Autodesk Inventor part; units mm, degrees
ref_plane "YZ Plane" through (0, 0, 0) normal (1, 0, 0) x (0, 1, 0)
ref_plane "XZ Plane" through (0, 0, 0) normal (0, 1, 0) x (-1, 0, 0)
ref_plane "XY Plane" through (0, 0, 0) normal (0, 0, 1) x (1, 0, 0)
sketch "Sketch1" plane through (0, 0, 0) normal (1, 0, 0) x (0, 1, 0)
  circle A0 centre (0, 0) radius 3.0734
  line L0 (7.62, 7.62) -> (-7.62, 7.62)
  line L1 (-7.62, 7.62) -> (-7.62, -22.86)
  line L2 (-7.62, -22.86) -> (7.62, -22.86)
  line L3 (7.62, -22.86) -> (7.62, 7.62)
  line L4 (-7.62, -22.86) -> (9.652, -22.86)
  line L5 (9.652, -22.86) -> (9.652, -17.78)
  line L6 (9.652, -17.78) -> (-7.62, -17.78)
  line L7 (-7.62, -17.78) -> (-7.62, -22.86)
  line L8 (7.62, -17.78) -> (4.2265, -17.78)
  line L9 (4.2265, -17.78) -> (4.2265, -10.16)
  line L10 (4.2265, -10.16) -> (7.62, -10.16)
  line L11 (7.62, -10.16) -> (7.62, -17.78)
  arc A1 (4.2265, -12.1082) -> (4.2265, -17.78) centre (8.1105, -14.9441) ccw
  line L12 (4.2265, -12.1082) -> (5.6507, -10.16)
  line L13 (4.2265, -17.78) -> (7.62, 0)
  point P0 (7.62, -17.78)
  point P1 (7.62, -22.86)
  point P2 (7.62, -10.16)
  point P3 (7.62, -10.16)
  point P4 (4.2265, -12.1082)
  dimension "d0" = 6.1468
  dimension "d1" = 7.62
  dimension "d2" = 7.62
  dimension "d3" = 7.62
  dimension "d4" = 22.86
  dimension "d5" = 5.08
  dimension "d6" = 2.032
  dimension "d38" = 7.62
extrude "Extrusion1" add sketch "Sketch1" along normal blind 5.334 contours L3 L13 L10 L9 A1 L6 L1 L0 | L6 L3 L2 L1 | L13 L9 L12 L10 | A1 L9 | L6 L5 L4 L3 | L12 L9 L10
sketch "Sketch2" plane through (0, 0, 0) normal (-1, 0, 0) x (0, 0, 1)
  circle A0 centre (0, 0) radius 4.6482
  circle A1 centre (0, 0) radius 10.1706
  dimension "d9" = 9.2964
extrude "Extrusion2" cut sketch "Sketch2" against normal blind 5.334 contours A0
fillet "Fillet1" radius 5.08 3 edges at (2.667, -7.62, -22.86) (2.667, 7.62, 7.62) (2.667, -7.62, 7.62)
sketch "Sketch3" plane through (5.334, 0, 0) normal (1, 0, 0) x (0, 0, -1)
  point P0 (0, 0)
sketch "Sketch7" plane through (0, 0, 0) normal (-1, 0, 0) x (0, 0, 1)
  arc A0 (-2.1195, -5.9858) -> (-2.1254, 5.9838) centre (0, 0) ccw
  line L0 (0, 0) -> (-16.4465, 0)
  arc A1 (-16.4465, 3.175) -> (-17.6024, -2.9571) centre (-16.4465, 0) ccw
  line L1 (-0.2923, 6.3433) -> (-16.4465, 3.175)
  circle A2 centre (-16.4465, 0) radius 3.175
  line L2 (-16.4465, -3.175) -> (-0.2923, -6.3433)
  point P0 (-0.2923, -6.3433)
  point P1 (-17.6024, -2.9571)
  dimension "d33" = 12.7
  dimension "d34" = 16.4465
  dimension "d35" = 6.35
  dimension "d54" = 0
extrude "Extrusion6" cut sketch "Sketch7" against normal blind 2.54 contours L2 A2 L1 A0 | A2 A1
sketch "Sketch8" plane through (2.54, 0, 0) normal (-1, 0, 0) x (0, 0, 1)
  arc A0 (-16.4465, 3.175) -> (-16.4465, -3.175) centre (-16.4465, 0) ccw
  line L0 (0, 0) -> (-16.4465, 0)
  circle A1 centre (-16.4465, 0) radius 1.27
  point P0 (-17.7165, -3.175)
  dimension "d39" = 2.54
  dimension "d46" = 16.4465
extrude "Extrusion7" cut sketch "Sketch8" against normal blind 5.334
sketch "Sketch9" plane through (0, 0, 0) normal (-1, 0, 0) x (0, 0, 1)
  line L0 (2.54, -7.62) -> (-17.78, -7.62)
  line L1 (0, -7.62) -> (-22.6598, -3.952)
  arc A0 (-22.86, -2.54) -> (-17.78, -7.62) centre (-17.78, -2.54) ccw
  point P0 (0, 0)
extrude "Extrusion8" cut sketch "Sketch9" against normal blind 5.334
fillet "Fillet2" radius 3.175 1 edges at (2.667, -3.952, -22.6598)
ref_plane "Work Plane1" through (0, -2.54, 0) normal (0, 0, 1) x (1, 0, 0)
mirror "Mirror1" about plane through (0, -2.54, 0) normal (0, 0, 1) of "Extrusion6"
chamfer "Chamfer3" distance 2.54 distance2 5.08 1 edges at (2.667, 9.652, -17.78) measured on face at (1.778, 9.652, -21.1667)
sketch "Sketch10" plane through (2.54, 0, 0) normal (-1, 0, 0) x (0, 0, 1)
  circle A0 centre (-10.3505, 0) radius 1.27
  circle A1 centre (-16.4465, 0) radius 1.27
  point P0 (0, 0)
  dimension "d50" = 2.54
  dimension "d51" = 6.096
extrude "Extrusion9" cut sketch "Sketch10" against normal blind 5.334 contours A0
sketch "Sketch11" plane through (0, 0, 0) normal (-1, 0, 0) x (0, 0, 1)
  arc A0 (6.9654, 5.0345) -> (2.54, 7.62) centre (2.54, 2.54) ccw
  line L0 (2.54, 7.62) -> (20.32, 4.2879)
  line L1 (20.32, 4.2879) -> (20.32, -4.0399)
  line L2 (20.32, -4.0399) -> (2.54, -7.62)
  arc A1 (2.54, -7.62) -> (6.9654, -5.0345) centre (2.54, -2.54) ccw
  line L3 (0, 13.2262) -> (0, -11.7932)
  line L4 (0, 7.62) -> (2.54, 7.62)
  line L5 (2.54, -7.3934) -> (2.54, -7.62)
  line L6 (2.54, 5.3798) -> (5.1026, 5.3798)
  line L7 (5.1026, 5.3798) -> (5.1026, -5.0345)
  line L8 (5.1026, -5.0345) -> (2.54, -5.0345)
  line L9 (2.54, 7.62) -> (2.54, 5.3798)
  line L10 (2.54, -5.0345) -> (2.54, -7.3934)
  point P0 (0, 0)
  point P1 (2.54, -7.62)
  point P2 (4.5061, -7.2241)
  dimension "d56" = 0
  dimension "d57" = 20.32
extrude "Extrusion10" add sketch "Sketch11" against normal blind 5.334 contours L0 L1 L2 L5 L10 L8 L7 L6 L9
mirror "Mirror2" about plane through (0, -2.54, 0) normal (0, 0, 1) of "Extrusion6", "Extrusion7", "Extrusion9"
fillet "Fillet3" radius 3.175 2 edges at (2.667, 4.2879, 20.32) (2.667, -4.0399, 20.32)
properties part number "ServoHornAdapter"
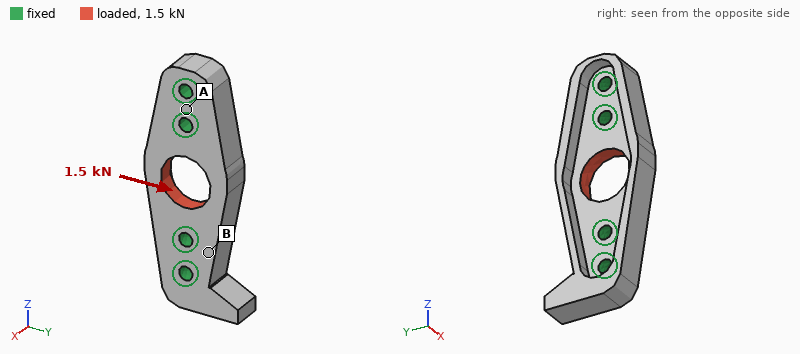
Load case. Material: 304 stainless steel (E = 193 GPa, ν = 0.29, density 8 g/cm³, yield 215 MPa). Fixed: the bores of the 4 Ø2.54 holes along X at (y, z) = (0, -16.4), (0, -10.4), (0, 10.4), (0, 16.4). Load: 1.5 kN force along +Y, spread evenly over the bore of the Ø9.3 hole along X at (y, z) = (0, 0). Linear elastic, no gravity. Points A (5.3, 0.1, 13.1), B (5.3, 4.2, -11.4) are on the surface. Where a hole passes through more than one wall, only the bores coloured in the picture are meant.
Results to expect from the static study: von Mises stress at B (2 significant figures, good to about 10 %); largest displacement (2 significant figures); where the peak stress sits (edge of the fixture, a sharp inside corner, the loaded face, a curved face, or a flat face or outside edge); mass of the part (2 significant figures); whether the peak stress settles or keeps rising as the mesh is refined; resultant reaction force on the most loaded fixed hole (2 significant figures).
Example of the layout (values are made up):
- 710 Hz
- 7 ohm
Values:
- 16 MPa
- 3.8 µm
- edge of the fixture
- 13 g
- keeps rising
- 850 N
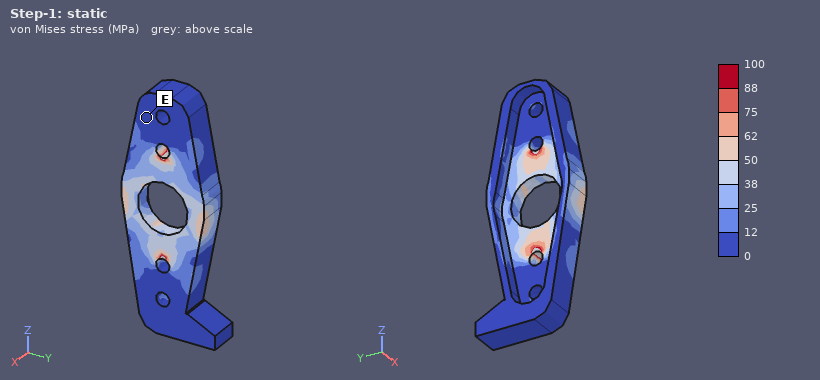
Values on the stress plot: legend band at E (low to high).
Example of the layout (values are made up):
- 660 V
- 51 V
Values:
- 0 to 12 MPa
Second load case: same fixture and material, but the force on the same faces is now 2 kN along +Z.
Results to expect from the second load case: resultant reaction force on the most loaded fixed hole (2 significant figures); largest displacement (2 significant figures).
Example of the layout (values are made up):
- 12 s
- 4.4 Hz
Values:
- 740 N
- 2.0 µm
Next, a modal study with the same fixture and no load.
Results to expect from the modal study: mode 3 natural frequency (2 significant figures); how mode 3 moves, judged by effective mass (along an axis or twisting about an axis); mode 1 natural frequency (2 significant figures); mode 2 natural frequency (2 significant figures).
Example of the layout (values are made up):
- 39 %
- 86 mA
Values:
- 27 kHz
- along X
- 24 kHz
- 24 kHz
